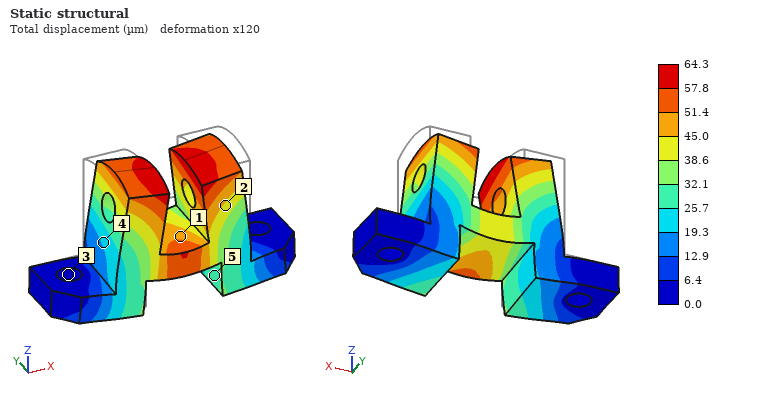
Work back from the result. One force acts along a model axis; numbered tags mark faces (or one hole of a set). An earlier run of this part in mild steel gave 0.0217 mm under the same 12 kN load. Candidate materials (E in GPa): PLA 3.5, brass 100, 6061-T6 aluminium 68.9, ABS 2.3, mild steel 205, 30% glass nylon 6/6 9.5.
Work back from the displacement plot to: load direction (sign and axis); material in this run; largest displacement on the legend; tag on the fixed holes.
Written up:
-Z
6061-T6 aluminium
64.3 µm
3
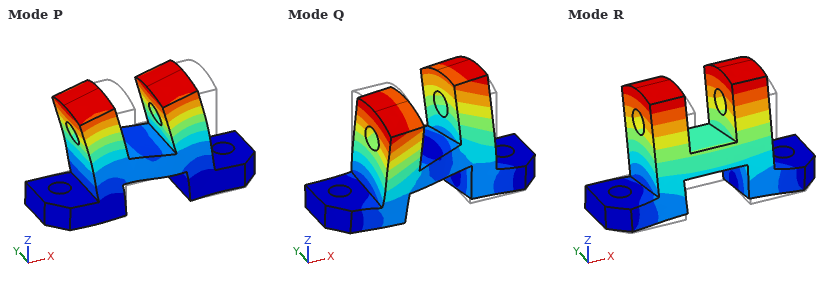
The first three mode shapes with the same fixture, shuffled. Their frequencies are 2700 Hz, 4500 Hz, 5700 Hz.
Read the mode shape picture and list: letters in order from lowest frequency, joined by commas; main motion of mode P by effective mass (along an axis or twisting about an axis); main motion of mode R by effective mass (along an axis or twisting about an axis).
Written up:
R, Q, P
along X
along Y
